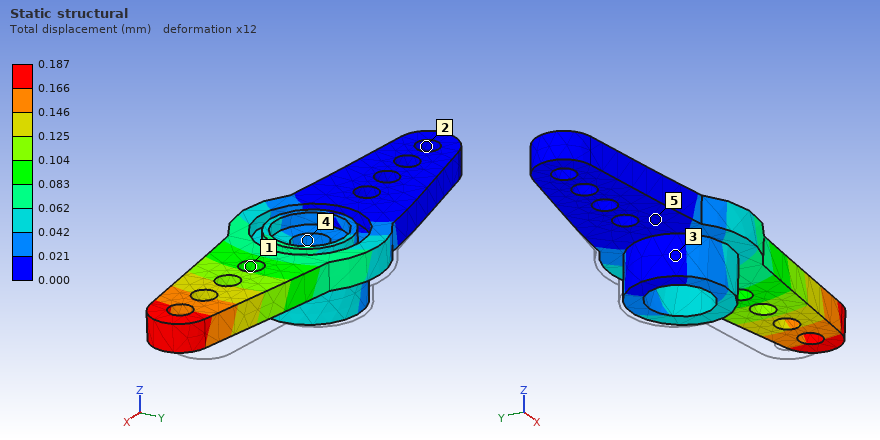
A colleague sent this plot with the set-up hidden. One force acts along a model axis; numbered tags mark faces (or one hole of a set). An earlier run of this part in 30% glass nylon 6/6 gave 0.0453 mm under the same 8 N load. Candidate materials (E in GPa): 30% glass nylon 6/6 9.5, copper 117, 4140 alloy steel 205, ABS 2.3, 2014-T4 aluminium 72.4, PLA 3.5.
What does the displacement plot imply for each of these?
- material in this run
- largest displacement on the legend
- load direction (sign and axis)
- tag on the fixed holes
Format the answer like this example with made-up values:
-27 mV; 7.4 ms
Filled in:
ABS; 0.187 mm; -Y; 2
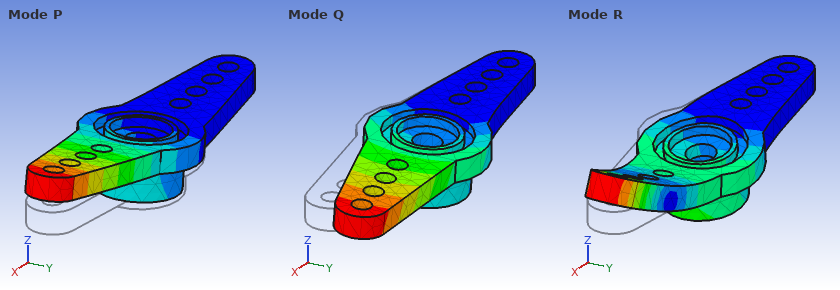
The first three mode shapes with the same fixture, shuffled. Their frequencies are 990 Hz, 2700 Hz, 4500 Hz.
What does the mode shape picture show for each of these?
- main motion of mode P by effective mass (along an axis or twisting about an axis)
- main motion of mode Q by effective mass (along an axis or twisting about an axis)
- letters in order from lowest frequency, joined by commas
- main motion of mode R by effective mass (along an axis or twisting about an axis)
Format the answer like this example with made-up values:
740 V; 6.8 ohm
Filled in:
along Z; along Y; P, Q, R; along Z
